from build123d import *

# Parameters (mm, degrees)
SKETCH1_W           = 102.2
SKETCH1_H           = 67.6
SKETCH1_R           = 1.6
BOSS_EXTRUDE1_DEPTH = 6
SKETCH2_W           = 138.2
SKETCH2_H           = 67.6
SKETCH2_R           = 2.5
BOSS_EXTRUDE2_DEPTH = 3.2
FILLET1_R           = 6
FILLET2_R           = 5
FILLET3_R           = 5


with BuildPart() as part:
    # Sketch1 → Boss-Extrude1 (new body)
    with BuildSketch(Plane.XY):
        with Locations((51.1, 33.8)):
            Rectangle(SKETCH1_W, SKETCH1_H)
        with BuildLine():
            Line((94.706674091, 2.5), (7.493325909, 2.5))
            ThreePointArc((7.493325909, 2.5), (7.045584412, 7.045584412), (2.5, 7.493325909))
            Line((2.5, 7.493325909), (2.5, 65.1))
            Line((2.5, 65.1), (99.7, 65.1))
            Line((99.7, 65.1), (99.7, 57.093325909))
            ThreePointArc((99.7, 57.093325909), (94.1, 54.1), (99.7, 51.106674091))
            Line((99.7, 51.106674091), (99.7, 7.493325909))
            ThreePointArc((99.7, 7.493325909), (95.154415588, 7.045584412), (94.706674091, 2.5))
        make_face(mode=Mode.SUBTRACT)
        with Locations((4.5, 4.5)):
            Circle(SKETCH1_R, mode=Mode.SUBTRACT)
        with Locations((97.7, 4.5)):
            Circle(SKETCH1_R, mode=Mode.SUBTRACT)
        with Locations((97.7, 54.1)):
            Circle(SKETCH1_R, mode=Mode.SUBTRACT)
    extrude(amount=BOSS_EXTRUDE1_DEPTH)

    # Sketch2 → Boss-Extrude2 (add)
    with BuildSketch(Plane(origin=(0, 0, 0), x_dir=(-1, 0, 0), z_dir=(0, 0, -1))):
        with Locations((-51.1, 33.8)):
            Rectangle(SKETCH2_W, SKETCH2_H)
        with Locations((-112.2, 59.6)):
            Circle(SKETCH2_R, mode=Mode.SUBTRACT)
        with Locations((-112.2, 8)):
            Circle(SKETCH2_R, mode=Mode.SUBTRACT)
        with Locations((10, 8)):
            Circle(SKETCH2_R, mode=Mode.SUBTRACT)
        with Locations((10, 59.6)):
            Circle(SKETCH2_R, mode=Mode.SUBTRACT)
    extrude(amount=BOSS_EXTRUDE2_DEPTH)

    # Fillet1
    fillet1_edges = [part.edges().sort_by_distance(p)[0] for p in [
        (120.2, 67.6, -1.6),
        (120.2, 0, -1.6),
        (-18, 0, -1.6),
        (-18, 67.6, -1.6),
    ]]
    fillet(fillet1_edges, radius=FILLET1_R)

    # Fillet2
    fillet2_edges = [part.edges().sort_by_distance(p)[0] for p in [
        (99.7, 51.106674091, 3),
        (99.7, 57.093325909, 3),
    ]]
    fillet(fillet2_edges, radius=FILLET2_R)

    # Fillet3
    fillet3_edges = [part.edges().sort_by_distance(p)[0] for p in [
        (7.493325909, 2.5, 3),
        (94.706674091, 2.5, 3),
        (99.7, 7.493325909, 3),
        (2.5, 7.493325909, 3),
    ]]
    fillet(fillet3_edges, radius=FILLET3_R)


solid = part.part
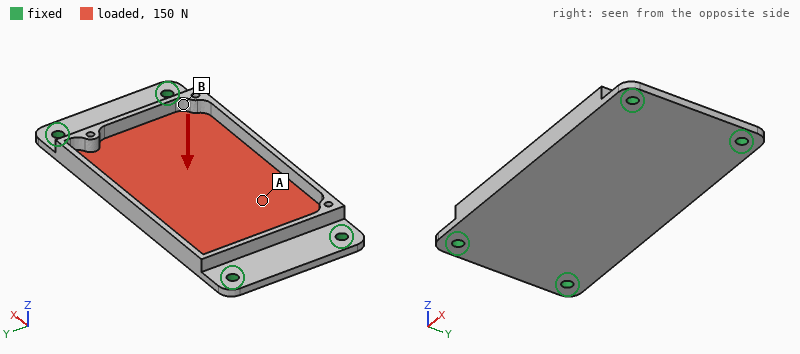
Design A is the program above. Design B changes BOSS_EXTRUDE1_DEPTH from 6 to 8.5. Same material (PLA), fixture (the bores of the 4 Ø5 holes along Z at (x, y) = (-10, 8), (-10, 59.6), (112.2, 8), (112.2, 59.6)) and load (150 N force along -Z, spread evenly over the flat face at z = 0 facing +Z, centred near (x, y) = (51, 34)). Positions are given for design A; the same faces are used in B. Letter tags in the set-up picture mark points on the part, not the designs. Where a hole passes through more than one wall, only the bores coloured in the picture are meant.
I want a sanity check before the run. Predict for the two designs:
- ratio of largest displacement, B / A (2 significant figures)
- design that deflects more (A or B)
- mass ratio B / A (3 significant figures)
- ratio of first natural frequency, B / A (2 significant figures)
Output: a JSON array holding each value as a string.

["0.74", "A", "1.07", "1.2"]
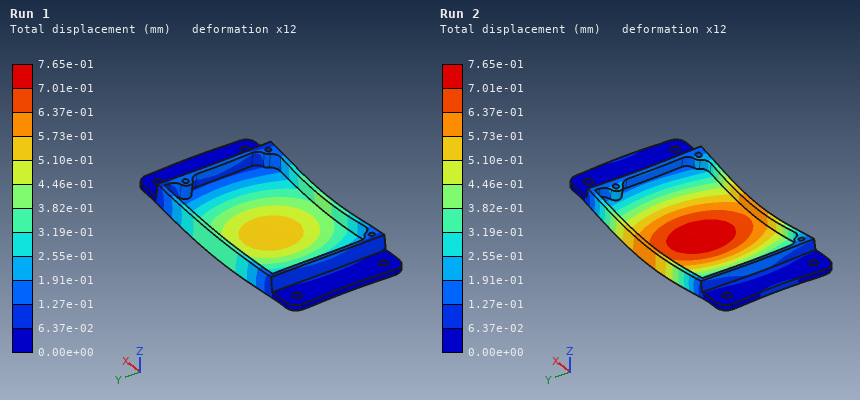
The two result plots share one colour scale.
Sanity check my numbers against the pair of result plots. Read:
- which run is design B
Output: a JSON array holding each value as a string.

["Run 1"]
